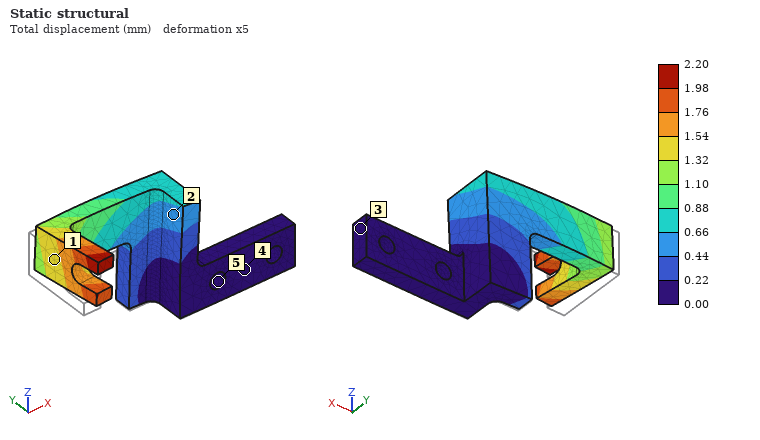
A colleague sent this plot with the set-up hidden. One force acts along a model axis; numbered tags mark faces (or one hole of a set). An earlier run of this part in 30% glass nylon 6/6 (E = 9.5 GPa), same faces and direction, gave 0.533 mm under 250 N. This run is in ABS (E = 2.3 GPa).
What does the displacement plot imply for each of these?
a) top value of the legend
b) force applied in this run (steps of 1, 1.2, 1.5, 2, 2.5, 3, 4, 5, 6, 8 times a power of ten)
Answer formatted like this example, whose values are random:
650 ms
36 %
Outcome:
2.20 mm
250 N
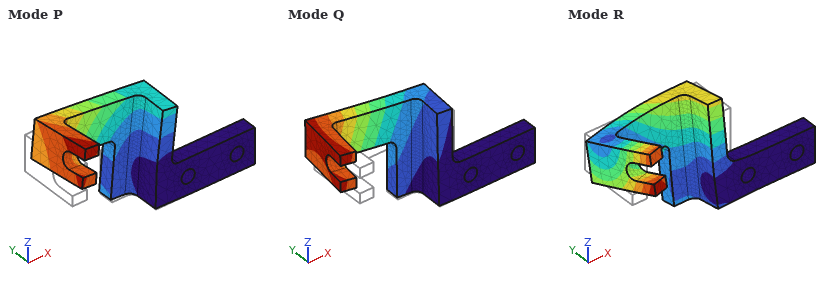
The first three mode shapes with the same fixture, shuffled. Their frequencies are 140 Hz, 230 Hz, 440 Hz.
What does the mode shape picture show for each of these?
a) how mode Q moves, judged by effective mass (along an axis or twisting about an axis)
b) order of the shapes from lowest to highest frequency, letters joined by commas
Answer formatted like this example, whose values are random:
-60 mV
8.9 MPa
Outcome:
along Y
Q, P, R
